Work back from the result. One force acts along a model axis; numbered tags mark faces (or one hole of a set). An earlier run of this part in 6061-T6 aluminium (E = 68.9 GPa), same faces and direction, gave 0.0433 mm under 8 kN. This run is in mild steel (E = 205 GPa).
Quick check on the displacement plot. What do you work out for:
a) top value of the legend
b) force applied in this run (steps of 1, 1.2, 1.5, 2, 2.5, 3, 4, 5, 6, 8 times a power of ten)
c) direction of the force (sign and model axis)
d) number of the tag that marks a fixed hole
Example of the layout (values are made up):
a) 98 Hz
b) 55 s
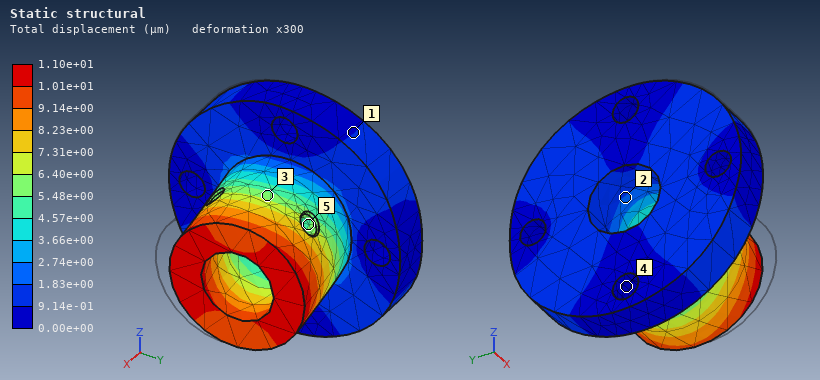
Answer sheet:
a) 1.10e+01 µm
b) 6 kN
c) +Y
d) 4
